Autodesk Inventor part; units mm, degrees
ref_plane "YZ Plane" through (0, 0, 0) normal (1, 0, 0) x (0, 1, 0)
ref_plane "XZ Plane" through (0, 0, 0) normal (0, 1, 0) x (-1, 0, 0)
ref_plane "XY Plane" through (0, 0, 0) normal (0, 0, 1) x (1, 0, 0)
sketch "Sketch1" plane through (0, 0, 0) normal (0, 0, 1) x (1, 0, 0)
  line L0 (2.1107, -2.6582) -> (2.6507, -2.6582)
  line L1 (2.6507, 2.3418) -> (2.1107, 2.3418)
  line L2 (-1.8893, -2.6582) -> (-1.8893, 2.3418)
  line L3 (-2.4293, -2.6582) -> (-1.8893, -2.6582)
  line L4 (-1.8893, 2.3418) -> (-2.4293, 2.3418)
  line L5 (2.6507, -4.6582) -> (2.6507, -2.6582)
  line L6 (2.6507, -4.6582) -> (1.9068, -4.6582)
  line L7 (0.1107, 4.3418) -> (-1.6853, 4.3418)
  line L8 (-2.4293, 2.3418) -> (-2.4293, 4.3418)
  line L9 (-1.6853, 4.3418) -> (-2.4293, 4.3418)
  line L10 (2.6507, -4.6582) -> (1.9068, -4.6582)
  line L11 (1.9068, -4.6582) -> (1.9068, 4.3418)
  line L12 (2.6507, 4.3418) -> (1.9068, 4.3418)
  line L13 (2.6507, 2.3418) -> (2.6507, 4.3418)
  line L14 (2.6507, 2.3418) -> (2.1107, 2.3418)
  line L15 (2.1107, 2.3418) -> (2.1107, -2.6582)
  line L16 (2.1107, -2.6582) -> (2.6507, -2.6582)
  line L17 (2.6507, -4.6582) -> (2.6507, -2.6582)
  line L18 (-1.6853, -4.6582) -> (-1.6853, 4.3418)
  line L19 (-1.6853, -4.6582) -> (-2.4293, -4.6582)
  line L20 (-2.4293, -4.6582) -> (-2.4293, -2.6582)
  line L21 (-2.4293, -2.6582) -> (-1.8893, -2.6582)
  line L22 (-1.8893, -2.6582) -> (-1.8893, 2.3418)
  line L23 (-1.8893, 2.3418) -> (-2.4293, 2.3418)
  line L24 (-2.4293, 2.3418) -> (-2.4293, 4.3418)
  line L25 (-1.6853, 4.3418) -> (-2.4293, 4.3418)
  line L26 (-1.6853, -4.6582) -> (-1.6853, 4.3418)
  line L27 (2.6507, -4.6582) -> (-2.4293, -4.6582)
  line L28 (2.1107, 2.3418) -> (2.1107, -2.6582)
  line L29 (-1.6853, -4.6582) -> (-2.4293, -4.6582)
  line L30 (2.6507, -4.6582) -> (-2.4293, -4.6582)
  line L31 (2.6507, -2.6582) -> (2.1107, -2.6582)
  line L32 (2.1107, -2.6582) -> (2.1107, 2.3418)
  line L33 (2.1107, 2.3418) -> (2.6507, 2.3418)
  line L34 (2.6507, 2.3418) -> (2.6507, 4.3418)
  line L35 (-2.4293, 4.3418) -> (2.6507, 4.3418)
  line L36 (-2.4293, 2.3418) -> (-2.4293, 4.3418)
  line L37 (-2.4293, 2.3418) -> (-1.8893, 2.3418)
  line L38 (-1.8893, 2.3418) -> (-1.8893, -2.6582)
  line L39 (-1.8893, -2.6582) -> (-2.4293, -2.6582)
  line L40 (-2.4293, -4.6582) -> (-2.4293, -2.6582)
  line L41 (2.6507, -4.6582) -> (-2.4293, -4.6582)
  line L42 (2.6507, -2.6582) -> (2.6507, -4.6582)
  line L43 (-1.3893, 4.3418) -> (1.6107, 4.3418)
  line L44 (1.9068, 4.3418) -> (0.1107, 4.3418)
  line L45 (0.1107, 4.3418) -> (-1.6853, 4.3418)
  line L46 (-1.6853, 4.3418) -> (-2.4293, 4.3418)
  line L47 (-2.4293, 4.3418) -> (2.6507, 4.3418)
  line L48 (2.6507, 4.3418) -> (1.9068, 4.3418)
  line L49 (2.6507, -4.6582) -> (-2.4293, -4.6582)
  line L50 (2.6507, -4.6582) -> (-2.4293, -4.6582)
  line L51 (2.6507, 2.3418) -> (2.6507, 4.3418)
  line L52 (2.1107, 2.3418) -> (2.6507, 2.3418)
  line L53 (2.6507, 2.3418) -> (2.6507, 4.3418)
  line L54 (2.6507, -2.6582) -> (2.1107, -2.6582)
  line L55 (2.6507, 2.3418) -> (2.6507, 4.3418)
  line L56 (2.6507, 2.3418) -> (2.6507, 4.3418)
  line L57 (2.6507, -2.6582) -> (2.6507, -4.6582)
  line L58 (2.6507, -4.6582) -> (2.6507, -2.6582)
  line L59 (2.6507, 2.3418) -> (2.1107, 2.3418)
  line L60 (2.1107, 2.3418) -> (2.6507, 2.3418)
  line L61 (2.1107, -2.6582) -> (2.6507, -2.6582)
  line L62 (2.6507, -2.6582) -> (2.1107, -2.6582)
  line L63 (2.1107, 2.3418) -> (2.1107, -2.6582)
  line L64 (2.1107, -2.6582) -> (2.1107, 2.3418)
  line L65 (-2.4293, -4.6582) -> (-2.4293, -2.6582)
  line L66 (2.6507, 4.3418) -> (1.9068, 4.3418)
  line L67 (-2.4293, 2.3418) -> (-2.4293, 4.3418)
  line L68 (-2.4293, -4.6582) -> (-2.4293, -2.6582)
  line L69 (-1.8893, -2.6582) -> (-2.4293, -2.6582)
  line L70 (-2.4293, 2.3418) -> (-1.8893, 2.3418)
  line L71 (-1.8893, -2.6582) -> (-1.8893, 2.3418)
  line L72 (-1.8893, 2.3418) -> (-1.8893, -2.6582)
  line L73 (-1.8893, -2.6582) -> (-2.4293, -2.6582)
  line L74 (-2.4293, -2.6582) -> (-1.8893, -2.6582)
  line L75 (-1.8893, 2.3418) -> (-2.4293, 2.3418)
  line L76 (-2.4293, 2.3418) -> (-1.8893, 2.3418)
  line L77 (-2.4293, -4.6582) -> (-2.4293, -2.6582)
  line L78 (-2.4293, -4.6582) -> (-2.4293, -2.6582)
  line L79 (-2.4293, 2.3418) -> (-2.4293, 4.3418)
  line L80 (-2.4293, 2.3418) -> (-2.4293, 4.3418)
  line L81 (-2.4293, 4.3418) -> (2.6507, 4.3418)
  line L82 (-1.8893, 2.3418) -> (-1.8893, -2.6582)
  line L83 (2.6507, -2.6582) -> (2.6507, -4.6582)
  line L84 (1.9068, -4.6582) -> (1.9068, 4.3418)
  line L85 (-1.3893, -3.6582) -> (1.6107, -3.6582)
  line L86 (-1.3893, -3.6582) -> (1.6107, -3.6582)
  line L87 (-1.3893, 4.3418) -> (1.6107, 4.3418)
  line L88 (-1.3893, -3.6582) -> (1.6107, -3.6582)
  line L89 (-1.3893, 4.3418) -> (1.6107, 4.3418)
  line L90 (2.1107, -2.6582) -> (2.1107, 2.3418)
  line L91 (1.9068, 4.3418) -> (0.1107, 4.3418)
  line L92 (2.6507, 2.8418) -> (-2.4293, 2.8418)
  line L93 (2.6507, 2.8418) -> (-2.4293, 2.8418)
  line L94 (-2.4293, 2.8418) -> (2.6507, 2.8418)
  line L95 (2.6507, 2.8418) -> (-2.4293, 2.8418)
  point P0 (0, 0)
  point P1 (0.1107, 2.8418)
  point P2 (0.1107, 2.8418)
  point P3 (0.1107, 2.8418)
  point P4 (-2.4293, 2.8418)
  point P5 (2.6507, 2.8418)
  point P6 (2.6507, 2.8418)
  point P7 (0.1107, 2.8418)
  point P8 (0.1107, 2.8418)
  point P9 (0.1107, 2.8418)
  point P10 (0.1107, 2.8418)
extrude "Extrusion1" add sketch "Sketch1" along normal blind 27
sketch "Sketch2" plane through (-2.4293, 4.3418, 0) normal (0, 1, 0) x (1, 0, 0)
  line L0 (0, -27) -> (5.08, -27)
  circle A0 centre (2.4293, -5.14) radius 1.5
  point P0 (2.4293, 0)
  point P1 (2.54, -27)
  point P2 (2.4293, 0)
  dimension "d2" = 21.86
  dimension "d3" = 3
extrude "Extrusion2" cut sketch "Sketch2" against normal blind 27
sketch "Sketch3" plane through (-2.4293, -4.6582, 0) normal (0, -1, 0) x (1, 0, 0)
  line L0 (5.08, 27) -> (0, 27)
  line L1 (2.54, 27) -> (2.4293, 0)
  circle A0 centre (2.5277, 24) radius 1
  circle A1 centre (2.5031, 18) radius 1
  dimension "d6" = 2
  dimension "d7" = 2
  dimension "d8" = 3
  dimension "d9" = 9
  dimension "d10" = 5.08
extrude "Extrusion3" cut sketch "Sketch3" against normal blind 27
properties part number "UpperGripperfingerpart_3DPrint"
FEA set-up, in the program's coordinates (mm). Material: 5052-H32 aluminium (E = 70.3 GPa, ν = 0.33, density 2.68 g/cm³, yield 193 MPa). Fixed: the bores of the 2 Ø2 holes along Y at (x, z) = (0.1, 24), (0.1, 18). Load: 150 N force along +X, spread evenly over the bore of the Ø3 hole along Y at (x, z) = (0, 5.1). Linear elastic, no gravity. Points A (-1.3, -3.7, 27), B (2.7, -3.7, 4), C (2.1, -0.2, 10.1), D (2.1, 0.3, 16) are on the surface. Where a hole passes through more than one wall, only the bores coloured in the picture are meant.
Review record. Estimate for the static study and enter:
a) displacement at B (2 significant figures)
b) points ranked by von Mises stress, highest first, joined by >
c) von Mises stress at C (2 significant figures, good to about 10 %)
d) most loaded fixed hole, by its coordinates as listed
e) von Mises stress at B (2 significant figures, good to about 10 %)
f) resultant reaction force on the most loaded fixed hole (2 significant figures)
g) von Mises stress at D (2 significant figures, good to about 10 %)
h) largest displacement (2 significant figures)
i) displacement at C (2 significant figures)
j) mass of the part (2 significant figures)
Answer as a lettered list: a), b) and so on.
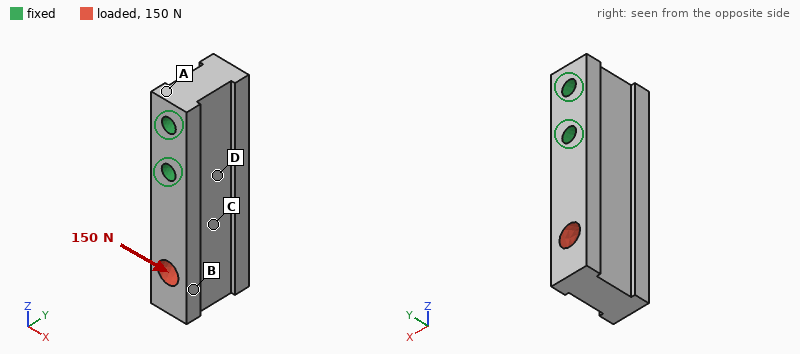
a) 32 µm
b) D > C > B > A
c) 21 MPa
d) (0.1, 18)
e) 13 MPa
f) 240 N
g) 46 MPa
h) 43 µm
i) 13 µm
j) 2.6 g
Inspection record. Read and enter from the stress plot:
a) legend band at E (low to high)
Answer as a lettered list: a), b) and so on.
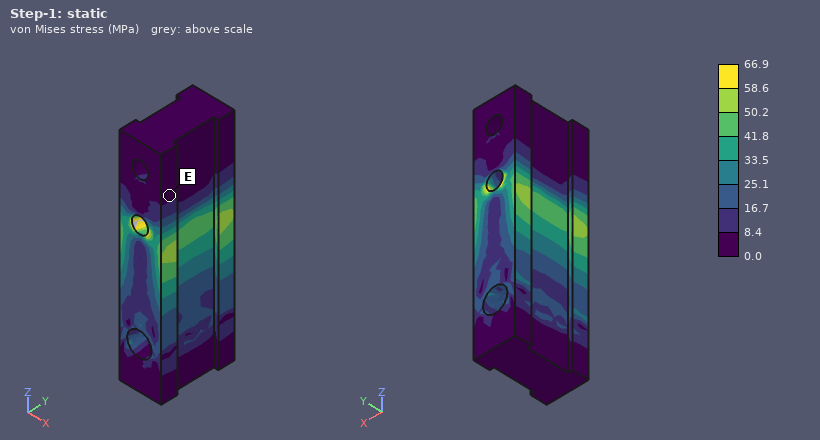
a) 0.0 to 8.4 MPa
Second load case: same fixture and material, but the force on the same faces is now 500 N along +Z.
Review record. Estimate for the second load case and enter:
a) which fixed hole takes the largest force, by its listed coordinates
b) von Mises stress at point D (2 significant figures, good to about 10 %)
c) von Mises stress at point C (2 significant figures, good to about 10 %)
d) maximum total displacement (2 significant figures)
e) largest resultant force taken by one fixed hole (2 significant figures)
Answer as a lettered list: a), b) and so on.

a) (0.1, 18)
b) 6.8 MPa
c) 12 MPa
d) 4.0 µm
e) 470 N
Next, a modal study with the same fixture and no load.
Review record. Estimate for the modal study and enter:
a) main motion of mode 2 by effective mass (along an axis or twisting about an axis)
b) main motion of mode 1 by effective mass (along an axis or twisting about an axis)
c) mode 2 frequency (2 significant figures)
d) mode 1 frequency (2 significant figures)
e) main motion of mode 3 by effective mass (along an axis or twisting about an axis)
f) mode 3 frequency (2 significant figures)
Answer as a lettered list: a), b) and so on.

a) along Y
b) along X
c) 21 kHz
d) 11 kHz
e) twisting about Z
f) 31 kHz
